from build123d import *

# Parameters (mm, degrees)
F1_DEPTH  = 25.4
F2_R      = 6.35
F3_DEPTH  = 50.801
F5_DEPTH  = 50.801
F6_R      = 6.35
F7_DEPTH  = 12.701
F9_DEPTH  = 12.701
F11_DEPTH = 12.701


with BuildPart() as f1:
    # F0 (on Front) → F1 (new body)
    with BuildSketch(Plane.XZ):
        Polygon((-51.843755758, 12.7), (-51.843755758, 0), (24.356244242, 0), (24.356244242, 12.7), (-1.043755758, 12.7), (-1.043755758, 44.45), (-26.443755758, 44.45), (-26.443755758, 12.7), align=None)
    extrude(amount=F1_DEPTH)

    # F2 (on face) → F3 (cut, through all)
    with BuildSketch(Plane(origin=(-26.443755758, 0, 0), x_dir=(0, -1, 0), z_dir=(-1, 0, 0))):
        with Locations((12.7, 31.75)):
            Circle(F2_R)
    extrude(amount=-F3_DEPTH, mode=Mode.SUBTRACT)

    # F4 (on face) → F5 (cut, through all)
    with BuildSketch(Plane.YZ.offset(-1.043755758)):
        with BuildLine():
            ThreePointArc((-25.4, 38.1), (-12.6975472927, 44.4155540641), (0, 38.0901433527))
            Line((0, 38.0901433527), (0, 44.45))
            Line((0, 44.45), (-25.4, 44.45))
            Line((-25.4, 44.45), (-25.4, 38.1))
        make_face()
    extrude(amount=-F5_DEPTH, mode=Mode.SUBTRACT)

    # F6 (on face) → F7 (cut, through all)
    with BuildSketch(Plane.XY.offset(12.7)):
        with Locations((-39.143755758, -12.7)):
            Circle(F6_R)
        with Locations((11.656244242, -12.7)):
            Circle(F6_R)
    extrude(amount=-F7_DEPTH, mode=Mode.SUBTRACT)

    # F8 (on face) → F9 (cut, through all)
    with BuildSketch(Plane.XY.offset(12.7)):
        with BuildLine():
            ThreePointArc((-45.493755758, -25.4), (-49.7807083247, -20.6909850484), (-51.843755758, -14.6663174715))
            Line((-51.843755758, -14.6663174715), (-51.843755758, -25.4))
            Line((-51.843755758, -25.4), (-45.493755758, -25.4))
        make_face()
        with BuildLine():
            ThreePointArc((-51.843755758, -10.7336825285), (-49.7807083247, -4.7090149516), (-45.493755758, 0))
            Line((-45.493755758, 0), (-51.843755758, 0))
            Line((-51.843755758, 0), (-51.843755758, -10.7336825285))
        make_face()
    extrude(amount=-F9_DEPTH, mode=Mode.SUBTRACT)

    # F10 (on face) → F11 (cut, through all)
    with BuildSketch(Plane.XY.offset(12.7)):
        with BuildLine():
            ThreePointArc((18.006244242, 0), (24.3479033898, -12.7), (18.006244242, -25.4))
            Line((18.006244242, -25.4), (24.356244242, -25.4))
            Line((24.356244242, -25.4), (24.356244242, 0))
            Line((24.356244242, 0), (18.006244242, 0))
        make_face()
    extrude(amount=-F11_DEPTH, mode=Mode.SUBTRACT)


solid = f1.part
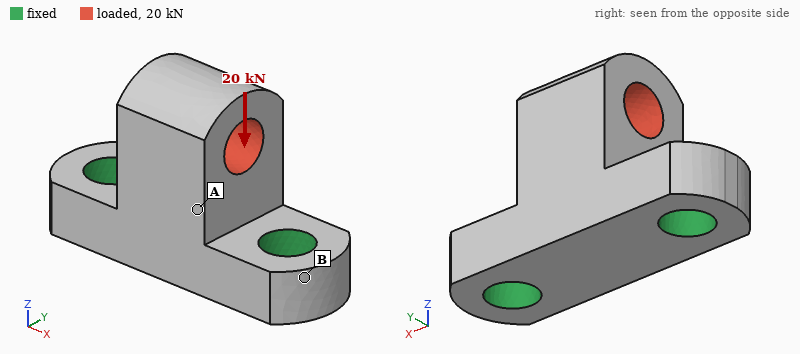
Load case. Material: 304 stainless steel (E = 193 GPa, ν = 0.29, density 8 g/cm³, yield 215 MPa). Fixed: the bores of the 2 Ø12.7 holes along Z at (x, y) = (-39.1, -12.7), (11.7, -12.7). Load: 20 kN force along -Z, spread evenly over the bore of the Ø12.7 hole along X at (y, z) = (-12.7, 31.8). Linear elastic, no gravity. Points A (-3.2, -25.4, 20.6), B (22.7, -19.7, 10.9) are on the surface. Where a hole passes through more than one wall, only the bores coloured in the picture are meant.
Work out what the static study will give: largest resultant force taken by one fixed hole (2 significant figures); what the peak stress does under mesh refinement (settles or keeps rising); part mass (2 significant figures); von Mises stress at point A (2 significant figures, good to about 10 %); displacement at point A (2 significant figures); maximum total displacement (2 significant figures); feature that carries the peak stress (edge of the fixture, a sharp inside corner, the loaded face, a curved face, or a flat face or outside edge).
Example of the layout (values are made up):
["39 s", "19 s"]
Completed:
["10 kN", "keeps rising", "290 g", "46 MPa", "10 µm", "16 µm", "edge of the fixture"]
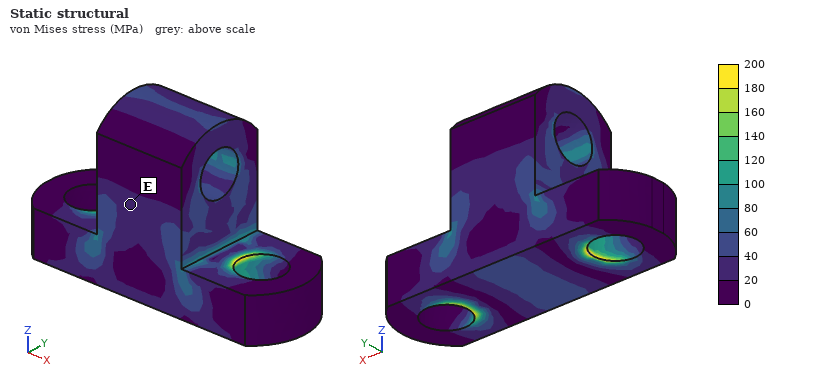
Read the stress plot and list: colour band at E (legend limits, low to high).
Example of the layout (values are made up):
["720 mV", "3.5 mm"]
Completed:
["20 to 40 MPa"]
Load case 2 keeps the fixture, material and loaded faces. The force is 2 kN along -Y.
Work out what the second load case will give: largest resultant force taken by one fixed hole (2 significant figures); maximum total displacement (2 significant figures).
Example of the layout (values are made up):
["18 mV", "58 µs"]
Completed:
["1.0 kN", "16 µm"]
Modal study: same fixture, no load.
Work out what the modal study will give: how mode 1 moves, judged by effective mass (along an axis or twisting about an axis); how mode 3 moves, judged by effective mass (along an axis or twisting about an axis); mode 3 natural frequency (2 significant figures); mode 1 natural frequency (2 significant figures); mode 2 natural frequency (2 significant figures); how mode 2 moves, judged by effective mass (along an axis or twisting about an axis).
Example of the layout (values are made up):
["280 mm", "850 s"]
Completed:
["along Y", "along Z", "16 kHz", "6600 Hz", "11 kHz", "along X"]
